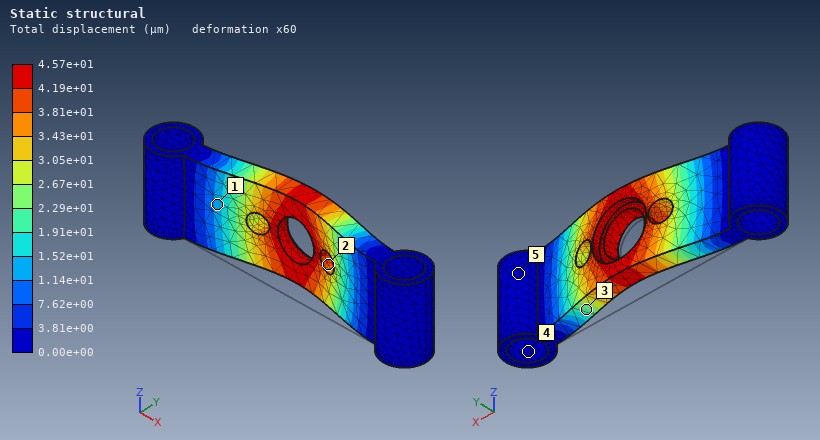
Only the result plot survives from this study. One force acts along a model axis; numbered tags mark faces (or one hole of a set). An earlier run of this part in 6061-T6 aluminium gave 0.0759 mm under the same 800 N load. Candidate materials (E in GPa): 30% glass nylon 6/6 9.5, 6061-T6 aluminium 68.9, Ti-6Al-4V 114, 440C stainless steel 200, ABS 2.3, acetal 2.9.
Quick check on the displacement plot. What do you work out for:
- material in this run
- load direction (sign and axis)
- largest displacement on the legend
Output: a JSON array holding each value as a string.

["Ti-6Al-4V", "+Y", "4.57e+01 µm"]
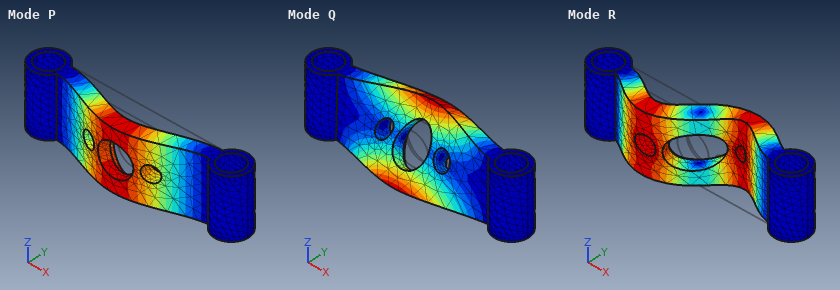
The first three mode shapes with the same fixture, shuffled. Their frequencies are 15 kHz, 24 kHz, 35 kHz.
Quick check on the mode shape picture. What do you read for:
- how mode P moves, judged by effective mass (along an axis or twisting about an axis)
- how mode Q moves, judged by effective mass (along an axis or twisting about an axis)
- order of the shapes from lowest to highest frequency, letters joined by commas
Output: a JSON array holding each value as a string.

["along Y", "twisting about X", "P, Q, R"]
